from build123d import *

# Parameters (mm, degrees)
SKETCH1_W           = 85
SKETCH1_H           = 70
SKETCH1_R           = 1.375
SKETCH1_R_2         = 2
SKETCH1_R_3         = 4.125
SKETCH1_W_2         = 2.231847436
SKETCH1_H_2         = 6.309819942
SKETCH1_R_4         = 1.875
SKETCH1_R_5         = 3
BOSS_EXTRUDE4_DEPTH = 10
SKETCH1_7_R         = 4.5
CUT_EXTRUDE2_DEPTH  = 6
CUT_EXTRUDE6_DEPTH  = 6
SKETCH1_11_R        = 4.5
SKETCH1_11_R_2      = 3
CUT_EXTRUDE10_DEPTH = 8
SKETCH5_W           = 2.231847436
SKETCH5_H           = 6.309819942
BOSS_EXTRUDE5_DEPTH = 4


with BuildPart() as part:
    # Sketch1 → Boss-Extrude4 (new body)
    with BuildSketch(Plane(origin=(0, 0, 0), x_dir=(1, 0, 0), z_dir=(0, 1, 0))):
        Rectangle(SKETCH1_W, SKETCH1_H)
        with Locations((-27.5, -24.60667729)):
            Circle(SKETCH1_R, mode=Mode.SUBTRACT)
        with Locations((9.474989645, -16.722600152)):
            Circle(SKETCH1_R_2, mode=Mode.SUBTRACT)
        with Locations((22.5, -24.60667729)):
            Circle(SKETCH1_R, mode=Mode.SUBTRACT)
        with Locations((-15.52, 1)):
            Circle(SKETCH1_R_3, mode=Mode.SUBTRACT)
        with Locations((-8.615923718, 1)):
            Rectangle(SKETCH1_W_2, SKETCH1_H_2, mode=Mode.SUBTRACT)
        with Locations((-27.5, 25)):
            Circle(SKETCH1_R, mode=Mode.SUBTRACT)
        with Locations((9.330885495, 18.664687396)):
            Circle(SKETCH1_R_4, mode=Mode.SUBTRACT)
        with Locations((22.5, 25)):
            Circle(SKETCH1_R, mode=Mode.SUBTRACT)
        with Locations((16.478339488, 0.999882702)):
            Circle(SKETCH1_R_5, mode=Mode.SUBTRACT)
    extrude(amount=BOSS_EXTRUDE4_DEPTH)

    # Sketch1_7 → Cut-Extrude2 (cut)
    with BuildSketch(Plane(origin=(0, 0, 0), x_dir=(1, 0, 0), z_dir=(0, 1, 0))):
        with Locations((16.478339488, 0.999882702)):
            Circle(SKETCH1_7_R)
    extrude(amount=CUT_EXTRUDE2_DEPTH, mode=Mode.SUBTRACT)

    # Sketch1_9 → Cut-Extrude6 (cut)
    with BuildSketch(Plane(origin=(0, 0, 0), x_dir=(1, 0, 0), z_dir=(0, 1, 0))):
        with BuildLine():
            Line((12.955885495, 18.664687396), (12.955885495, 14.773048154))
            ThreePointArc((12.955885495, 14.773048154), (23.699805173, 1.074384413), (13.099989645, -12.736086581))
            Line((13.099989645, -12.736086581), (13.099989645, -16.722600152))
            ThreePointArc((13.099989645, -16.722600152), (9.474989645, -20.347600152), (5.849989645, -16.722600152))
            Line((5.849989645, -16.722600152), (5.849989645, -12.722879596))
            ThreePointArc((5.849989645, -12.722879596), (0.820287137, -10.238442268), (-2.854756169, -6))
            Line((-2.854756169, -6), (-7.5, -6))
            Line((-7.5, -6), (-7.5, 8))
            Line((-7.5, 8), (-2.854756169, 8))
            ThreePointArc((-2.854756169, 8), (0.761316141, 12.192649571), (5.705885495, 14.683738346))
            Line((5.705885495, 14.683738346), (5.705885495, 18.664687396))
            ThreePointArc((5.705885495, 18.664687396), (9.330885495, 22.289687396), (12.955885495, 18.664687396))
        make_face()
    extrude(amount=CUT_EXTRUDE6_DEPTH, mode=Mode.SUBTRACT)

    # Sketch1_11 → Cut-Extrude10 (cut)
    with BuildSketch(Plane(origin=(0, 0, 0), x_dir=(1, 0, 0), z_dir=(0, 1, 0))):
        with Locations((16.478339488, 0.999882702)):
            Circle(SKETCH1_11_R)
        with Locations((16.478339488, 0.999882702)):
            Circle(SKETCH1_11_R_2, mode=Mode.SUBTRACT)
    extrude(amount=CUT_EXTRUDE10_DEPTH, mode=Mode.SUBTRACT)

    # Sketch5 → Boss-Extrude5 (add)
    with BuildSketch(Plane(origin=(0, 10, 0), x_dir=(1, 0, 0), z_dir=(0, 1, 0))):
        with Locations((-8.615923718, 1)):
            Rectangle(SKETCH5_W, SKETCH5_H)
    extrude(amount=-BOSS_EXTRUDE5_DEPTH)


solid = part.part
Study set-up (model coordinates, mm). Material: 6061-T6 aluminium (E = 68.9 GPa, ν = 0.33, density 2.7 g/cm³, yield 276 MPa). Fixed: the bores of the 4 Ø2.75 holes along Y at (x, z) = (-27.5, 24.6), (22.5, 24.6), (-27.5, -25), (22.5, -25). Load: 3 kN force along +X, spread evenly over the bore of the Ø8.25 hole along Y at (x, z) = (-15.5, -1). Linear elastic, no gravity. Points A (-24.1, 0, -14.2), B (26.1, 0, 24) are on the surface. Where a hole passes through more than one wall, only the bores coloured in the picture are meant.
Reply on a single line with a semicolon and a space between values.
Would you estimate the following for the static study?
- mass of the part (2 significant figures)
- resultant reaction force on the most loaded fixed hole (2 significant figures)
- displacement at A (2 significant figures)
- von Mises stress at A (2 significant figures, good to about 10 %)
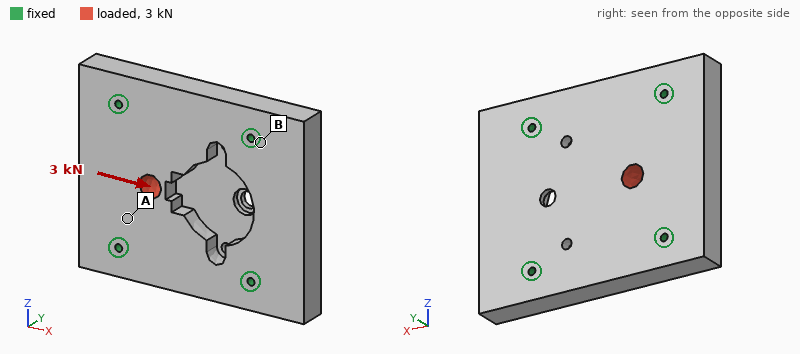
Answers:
150 g; 1.0 kN; 2.4 µm; 6.3 MPa
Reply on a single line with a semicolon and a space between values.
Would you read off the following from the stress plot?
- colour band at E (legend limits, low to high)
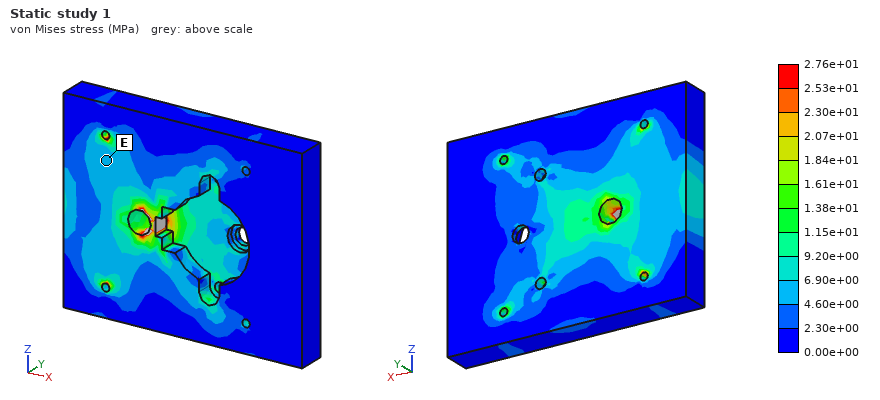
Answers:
4.60e+00 to 6.90e+00 MPa
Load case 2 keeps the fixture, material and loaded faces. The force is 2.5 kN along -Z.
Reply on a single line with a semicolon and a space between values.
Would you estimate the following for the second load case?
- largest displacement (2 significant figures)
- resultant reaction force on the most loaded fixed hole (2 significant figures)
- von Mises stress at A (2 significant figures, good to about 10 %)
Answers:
3.5 µm; 1.0 kN; 6.8 MPa
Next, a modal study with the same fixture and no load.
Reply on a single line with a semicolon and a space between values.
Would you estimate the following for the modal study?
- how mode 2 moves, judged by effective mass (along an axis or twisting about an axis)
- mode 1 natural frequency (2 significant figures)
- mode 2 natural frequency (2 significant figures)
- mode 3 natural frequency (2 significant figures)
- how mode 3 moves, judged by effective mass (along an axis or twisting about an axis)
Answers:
along Y; 9900 Hz; 11 kHz; 13 kHz; twisting about Z
